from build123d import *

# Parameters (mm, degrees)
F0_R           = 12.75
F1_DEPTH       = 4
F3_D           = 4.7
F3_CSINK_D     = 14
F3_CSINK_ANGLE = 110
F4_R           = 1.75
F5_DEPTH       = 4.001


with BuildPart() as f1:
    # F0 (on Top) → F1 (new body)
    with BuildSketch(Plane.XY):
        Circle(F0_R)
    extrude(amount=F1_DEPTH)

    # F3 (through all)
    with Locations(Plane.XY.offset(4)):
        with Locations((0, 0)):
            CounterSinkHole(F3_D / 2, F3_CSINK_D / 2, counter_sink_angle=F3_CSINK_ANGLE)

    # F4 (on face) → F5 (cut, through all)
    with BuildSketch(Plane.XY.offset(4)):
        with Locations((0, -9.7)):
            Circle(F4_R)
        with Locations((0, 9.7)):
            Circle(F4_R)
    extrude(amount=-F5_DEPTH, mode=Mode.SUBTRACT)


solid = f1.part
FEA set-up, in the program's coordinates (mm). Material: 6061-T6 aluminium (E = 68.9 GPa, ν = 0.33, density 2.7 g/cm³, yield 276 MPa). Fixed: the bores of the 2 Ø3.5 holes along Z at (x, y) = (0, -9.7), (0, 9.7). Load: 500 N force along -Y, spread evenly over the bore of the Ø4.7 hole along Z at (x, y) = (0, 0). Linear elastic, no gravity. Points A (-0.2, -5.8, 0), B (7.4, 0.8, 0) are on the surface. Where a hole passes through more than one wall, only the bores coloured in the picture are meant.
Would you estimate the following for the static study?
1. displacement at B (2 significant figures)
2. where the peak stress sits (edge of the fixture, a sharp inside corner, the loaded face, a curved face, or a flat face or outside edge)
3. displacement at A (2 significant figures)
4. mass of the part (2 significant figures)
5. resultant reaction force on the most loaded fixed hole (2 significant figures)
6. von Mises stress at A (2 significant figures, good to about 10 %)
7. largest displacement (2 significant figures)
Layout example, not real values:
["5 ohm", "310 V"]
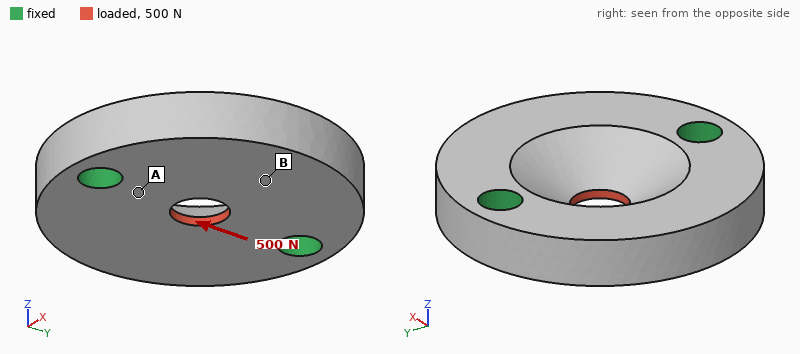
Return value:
["0.60 µm", "the loaded face", "0.63 µm", "4.6 g", "250 N", "23 MPa", "3.1 µm"]
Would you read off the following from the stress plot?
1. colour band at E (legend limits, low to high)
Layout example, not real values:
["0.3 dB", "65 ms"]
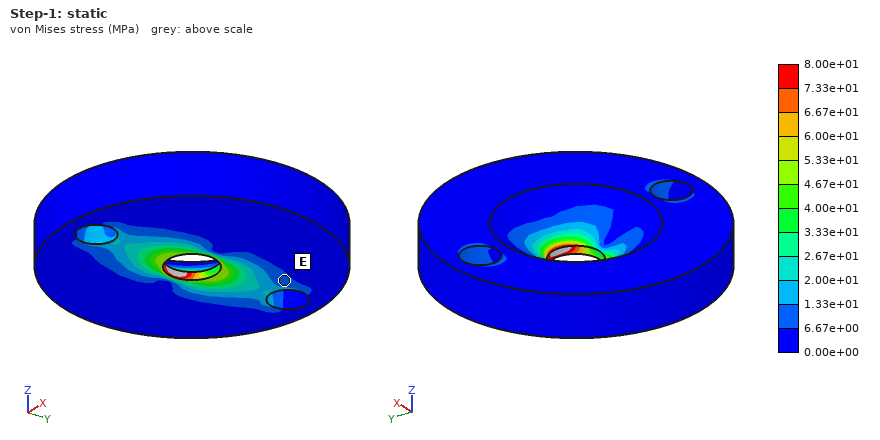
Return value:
["6.67e+00 to 1.33e+01 MPa"]
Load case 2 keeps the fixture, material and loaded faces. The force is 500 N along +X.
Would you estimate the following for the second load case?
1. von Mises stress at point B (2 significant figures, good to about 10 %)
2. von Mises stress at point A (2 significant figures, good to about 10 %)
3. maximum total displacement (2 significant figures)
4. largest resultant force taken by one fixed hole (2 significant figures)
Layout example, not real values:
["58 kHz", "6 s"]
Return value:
["6.9 MPa", "8.0 MPa", "4.0 µm", "250 N"]
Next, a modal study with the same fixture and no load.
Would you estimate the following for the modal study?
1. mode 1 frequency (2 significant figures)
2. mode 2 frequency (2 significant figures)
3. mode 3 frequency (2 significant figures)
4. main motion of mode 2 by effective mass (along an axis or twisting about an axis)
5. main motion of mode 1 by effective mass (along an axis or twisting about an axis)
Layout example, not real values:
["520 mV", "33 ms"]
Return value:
["19 kHz", "21 kHz", "46 kHz", "along Z", "twisting about Y"]
